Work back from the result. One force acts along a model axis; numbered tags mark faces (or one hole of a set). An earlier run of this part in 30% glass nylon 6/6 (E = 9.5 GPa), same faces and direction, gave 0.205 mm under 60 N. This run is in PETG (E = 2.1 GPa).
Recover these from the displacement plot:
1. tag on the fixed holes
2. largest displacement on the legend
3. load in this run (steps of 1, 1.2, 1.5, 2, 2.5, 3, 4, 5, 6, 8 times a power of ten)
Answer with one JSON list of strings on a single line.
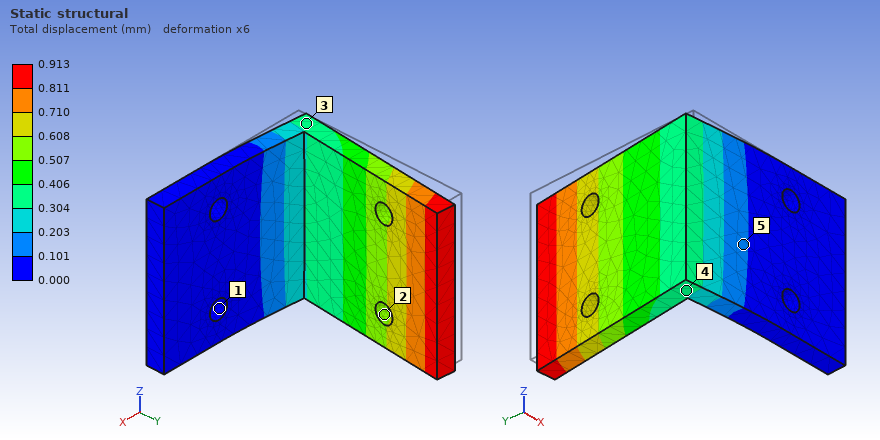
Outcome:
["1", "0.913 mm", "60 N"]
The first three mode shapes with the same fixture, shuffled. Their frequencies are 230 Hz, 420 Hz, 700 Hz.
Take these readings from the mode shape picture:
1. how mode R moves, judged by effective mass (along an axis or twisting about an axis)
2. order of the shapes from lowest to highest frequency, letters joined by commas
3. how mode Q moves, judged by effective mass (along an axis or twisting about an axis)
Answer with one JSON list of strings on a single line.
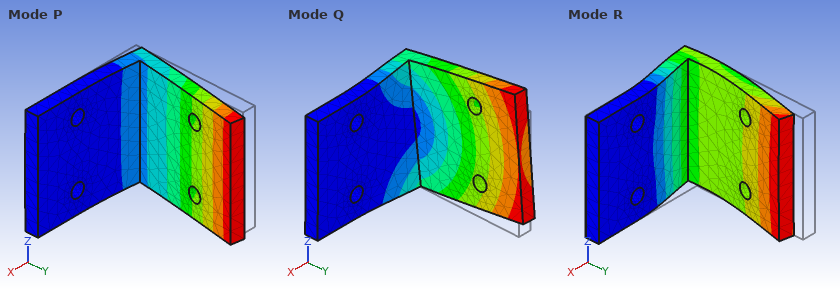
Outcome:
["along Y", "P, Q, R", "along Z"]
